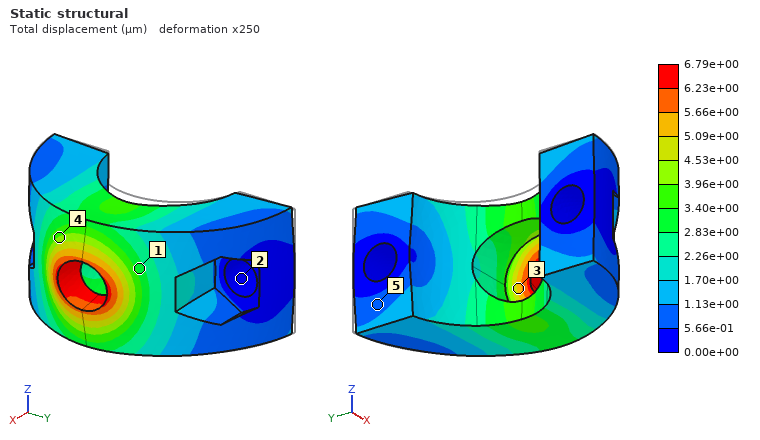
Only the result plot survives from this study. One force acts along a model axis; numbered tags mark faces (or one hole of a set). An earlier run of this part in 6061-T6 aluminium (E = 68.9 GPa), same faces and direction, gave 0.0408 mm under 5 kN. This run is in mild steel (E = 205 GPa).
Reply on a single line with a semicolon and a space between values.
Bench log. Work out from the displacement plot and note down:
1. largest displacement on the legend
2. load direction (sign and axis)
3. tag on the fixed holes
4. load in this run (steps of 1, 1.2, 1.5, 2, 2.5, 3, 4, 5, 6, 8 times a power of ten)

6.79e+00 µm; +X; 2; 2.5 kN
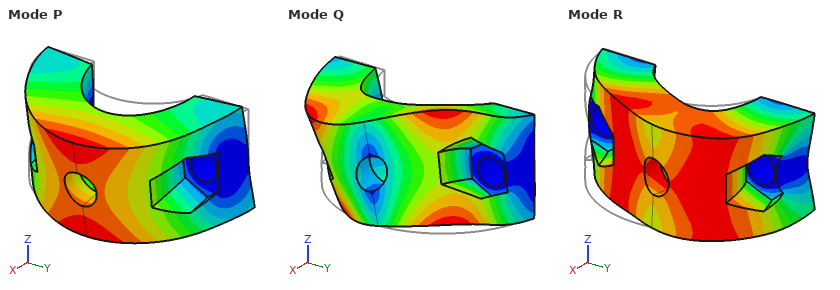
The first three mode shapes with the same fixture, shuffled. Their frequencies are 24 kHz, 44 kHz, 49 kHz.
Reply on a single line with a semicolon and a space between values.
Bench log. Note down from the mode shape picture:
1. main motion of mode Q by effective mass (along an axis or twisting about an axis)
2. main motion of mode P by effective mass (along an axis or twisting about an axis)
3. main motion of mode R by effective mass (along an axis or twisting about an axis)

twisting about X; along Z; along Y
